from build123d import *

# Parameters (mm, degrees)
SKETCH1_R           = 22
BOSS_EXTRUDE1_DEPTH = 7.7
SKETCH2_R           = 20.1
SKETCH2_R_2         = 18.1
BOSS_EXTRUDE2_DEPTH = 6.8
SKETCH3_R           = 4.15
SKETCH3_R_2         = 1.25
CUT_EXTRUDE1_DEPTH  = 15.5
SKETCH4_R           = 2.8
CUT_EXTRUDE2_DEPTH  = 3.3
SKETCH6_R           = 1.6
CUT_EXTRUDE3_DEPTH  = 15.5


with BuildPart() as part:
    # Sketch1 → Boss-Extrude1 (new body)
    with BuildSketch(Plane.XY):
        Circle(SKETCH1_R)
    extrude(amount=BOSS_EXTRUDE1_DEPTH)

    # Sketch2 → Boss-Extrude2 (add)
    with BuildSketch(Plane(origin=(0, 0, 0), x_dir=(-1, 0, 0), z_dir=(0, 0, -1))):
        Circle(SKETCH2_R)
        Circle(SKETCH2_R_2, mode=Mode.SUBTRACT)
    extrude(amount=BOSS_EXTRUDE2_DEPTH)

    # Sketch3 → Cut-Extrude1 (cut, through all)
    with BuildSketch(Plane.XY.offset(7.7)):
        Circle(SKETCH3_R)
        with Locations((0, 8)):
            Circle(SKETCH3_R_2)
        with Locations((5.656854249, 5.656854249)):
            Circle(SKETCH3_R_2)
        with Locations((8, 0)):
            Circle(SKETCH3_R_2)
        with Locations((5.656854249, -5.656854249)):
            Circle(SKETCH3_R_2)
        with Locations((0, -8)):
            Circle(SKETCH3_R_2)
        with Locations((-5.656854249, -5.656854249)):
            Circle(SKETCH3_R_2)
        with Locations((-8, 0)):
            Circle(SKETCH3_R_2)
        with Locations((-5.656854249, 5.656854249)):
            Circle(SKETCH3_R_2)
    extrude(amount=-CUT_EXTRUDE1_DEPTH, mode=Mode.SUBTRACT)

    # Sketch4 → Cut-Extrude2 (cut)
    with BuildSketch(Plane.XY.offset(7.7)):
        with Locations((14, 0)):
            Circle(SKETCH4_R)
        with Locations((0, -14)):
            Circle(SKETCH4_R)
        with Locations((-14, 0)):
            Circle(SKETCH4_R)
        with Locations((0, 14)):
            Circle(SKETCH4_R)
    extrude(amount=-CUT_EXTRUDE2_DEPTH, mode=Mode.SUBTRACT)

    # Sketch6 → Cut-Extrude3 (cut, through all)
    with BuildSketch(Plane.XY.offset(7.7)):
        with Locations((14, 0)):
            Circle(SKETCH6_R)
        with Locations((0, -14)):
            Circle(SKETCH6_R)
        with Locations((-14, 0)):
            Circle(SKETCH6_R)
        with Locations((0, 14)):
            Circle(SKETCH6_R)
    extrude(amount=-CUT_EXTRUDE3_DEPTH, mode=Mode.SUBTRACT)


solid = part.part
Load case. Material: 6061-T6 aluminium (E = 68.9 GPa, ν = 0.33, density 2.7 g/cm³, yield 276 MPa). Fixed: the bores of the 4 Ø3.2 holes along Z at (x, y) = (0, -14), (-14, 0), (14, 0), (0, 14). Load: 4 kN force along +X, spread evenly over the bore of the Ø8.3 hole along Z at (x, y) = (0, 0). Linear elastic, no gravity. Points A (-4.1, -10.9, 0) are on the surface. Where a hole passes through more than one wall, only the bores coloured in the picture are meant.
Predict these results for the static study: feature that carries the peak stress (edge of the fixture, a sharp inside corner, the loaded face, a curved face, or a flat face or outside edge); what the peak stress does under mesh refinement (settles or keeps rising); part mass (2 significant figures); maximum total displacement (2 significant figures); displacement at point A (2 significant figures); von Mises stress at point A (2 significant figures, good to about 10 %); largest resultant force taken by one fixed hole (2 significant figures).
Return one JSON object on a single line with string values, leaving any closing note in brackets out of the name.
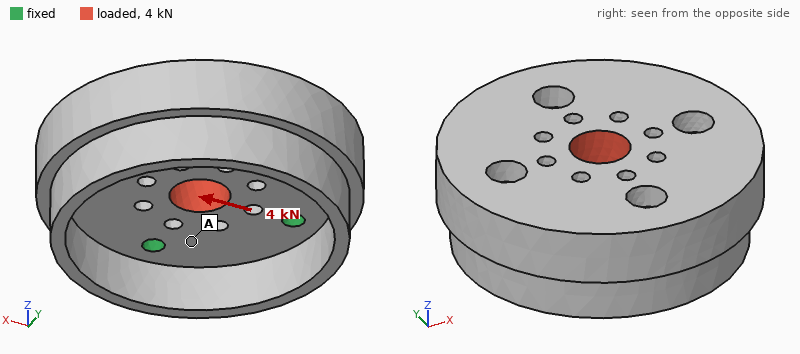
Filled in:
{"feature that carries the peak stress": "edge of the fixture", "what the peak stress does under mesh refinement": "keeps rising", "part mass": "33 g", "maximum total displacement": "4.8 µm", "displacement at point A": "1.1 µm", "von Mises stress at point A": "10 MPa", "largest resultant force taken by one fixed hole": "1.2 kN"}
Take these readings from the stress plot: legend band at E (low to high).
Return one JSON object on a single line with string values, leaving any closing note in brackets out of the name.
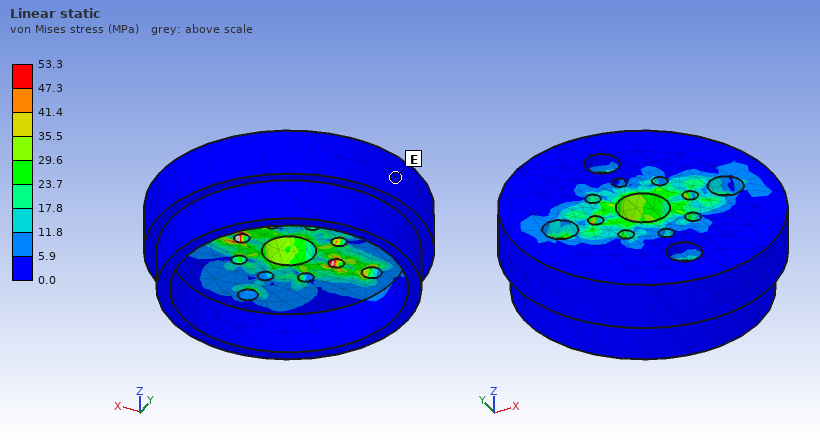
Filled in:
{"legend band at E": "0.0 to 5.9 MPa"}
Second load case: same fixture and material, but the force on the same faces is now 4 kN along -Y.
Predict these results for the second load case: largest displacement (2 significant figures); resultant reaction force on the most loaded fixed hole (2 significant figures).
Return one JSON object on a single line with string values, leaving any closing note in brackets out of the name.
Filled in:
{"largest displacement": "4.8 µm", "resultant reaction force on the most loaded fixed hole": "1.2 kN"}
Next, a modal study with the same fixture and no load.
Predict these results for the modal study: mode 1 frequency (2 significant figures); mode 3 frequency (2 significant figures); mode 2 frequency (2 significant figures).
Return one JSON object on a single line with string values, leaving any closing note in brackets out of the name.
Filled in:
{"mode 1 frequency": "20 kHz", "mode 3 frequency": "25 kHz", "mode 2 frequency": "25 kHz"}
